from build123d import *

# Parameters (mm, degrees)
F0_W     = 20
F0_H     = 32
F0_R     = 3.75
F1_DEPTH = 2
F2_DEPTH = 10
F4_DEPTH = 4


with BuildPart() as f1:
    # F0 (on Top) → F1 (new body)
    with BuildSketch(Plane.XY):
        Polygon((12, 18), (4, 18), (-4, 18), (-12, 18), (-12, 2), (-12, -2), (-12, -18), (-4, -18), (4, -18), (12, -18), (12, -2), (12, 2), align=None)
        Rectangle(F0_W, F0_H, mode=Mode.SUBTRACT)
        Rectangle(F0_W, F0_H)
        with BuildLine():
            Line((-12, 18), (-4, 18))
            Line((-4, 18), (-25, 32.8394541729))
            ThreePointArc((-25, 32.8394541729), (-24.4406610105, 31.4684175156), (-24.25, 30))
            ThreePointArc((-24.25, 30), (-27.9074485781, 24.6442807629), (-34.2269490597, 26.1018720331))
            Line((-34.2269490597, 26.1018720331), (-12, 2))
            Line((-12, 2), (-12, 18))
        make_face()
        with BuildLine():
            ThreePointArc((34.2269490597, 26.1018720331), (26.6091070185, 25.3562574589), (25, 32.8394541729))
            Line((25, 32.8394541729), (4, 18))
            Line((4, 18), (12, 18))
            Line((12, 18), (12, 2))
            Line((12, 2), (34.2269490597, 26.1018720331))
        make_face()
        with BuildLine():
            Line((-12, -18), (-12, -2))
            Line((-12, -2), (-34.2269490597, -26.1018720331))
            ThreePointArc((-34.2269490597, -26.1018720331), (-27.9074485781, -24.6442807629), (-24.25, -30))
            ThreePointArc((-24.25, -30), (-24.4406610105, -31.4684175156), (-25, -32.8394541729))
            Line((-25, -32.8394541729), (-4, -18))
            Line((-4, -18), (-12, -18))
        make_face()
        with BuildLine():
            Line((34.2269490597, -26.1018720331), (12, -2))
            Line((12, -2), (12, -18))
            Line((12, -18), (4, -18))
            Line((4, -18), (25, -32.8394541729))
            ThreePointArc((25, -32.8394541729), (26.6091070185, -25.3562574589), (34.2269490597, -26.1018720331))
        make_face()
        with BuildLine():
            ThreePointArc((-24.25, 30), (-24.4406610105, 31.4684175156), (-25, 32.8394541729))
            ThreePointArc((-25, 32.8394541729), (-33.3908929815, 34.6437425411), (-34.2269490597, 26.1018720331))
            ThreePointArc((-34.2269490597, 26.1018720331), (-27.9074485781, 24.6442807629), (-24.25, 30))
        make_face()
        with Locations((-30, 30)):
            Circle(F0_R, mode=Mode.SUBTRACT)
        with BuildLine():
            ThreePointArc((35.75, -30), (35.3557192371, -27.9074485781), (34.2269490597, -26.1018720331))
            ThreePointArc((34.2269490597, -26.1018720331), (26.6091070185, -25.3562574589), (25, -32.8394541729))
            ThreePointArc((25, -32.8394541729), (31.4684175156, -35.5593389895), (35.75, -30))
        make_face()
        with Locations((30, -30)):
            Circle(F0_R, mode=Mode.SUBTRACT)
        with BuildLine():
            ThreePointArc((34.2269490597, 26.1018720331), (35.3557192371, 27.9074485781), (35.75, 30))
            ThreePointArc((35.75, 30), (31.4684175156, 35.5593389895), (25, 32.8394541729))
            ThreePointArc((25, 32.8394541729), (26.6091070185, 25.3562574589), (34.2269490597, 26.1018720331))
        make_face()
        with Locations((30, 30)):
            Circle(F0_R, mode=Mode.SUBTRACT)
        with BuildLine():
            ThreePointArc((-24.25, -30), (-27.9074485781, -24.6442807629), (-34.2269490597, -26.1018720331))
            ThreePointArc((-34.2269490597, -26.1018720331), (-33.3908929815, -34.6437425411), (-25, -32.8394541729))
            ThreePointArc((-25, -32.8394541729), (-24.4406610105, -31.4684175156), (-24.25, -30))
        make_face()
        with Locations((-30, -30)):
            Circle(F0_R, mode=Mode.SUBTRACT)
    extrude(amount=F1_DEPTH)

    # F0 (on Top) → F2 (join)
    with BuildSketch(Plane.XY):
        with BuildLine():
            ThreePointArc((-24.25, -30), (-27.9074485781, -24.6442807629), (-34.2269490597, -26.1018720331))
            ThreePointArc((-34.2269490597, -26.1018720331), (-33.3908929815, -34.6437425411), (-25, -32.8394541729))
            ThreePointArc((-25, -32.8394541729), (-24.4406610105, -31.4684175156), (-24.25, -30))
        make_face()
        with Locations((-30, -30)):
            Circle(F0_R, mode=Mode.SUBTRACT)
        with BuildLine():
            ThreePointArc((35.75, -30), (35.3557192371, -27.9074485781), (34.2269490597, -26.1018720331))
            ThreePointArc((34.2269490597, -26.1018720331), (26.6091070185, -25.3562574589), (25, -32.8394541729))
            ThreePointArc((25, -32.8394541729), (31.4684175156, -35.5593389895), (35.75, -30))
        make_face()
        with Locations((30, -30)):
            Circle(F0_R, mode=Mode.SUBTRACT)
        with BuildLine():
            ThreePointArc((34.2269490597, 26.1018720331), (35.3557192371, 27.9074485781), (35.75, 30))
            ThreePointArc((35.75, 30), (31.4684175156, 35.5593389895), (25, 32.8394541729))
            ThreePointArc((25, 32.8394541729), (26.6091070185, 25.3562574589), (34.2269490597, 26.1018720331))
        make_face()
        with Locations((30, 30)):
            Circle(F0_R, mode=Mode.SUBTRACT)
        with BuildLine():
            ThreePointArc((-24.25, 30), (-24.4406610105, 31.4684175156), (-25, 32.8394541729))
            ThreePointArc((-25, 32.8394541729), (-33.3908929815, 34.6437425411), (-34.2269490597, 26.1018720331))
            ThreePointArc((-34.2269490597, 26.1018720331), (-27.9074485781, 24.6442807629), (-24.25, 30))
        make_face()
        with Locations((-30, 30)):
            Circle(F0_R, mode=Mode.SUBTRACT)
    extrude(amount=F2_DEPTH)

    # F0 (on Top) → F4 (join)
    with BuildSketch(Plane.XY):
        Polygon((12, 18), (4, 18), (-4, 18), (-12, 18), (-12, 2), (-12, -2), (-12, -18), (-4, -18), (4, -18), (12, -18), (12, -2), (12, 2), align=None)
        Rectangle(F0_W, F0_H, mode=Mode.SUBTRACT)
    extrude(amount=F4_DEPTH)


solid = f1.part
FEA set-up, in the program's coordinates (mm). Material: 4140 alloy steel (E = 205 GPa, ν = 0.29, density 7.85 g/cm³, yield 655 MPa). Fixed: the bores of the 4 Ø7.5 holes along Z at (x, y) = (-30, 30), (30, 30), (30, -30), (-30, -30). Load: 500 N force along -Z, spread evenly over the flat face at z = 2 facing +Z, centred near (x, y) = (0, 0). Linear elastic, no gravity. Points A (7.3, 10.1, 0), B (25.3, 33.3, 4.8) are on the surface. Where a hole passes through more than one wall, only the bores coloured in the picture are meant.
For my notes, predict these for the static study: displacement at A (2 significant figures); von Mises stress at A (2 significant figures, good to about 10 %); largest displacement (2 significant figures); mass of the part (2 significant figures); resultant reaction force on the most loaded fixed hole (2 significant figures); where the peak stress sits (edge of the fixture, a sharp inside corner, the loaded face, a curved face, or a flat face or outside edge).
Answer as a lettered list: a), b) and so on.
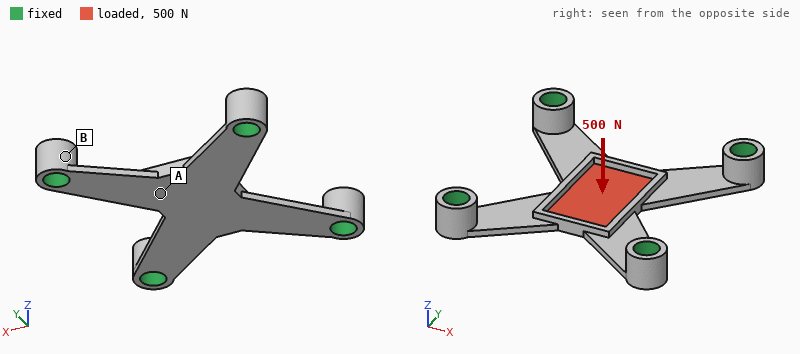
a) 0.099 mm
b) 57 MPa
c) 0.12 mm
d) 55 g
e) 170 N
f) a flat face or outside edge
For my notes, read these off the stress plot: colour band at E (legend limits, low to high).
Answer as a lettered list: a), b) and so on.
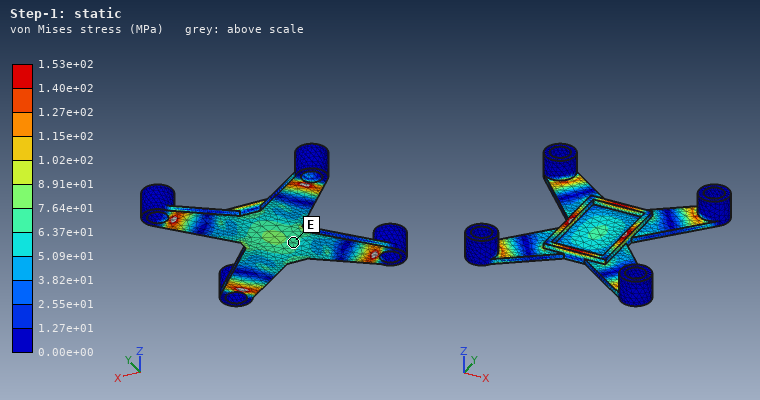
a) 6.37e+01 to 7.64e+01 MPa
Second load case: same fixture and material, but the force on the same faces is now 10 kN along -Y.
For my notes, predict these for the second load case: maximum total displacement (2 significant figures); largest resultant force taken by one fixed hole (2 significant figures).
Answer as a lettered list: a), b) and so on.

a) 68 µm
b) 3.3 kN
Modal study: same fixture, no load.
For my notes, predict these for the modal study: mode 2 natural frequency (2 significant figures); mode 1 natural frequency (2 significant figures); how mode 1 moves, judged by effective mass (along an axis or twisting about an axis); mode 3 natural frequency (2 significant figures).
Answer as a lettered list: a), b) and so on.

a) 5000 Hz
b) 2500 Hz
c) along Z
d) 5500 Hz
